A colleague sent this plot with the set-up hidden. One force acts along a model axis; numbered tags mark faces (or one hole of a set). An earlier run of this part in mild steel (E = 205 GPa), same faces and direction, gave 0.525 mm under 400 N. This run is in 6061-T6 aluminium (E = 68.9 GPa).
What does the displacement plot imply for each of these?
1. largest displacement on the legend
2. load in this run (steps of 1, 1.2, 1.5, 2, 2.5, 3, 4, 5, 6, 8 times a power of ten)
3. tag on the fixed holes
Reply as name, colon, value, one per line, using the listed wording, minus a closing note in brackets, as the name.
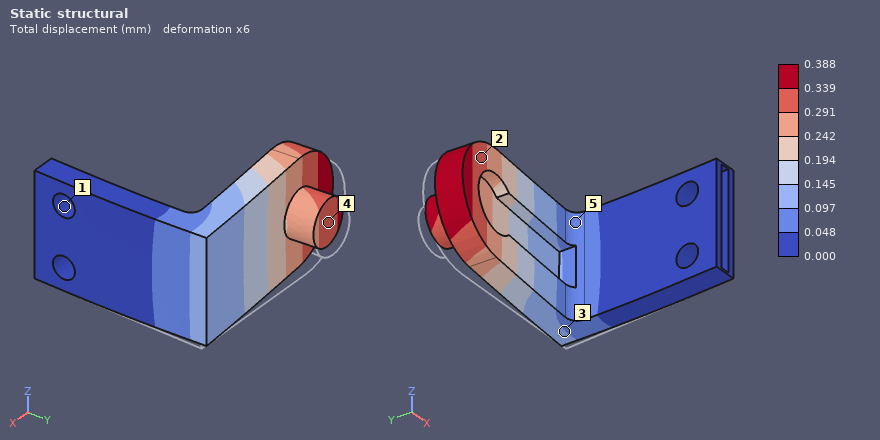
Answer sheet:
largest displacement on the legend: 0.388 mm
load in this run: 100 N
tag on the fixed holes: 1
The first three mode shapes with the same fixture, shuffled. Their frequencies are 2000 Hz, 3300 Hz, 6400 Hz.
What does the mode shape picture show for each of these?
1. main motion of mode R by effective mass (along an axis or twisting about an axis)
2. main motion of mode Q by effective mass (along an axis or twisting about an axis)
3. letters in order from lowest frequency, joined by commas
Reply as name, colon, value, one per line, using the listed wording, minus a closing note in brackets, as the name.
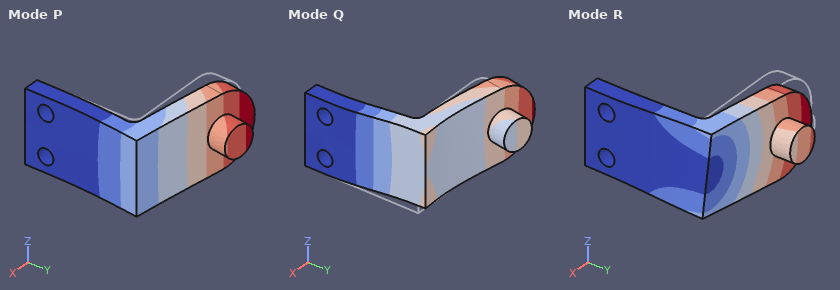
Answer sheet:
main motion of mode R by effective mass: along Z
main motion of mode Q by effective mass: along X
letters in order from lowest frequency, joined by commas: P, R, Q
